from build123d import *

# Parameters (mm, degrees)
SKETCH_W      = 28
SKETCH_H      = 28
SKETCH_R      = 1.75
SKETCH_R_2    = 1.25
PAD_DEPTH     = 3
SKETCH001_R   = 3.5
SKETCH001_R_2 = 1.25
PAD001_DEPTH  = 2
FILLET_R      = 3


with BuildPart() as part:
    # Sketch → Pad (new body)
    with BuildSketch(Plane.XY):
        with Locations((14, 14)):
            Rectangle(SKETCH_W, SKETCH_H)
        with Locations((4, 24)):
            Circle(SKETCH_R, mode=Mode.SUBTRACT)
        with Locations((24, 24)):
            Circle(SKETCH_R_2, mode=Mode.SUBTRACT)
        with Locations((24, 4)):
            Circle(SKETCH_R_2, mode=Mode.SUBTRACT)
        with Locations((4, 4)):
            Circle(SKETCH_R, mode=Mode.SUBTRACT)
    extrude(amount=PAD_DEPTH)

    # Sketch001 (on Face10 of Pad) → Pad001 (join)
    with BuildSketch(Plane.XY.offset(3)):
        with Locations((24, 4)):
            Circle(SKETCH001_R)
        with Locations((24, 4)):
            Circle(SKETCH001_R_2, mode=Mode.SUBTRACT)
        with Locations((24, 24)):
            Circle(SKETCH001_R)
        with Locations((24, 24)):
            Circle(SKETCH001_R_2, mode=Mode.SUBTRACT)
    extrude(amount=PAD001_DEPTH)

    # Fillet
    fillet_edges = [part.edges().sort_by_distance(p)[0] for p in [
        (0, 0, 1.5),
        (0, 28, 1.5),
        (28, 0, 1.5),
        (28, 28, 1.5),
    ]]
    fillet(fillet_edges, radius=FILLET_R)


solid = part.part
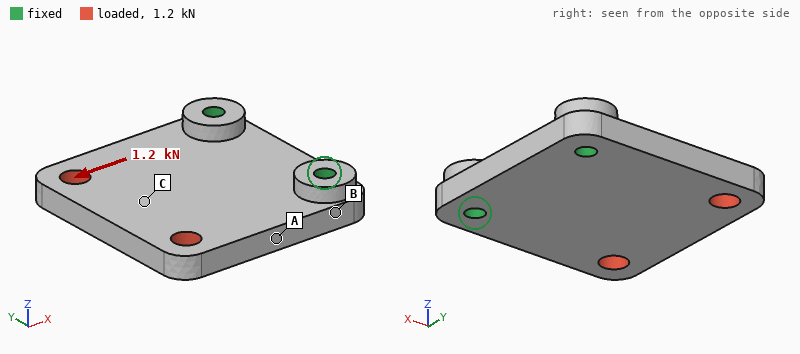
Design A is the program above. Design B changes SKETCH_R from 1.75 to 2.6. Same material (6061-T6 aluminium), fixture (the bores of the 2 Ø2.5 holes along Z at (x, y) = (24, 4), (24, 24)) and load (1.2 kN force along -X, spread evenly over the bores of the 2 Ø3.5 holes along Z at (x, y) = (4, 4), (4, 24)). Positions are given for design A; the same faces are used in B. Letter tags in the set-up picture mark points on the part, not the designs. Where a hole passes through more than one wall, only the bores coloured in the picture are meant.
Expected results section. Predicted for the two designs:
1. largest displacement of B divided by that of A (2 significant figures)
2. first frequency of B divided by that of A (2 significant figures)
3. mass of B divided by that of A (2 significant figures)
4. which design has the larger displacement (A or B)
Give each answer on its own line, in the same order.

1.3
1.0
0.97
B
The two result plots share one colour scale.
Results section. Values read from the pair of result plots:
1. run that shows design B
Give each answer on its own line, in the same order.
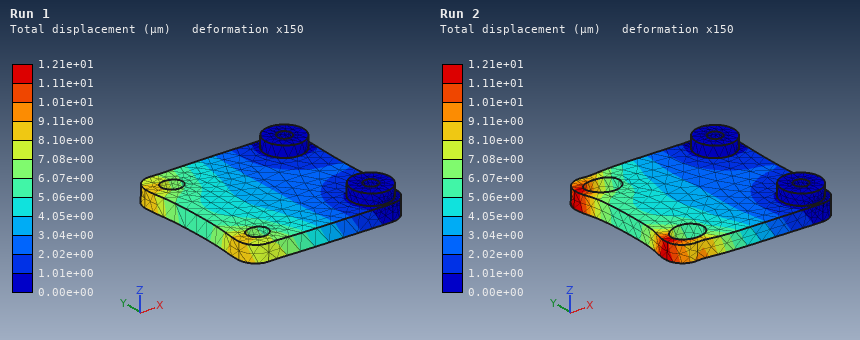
Run 2
